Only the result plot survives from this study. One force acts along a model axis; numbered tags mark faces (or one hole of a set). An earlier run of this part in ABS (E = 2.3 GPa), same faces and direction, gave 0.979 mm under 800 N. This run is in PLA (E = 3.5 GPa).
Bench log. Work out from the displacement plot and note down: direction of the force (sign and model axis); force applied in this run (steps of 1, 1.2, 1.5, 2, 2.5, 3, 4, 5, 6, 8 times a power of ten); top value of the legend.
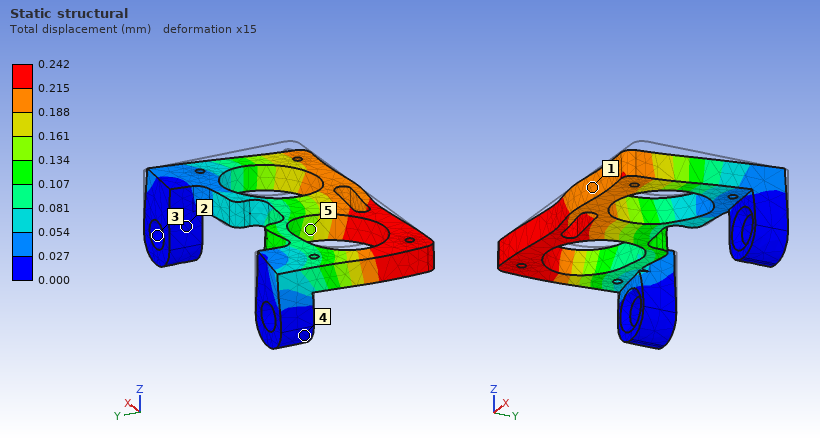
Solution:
-X
300 N
0.242 mm
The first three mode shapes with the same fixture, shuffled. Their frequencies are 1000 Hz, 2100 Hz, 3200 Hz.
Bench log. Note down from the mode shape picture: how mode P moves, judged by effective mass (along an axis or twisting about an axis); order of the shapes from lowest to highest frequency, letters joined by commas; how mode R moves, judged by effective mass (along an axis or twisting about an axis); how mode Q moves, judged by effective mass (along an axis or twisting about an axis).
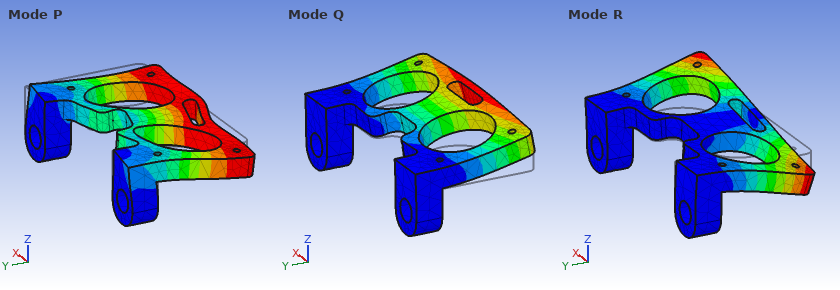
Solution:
along X
Q, R, P
twisting about Y
along Z
